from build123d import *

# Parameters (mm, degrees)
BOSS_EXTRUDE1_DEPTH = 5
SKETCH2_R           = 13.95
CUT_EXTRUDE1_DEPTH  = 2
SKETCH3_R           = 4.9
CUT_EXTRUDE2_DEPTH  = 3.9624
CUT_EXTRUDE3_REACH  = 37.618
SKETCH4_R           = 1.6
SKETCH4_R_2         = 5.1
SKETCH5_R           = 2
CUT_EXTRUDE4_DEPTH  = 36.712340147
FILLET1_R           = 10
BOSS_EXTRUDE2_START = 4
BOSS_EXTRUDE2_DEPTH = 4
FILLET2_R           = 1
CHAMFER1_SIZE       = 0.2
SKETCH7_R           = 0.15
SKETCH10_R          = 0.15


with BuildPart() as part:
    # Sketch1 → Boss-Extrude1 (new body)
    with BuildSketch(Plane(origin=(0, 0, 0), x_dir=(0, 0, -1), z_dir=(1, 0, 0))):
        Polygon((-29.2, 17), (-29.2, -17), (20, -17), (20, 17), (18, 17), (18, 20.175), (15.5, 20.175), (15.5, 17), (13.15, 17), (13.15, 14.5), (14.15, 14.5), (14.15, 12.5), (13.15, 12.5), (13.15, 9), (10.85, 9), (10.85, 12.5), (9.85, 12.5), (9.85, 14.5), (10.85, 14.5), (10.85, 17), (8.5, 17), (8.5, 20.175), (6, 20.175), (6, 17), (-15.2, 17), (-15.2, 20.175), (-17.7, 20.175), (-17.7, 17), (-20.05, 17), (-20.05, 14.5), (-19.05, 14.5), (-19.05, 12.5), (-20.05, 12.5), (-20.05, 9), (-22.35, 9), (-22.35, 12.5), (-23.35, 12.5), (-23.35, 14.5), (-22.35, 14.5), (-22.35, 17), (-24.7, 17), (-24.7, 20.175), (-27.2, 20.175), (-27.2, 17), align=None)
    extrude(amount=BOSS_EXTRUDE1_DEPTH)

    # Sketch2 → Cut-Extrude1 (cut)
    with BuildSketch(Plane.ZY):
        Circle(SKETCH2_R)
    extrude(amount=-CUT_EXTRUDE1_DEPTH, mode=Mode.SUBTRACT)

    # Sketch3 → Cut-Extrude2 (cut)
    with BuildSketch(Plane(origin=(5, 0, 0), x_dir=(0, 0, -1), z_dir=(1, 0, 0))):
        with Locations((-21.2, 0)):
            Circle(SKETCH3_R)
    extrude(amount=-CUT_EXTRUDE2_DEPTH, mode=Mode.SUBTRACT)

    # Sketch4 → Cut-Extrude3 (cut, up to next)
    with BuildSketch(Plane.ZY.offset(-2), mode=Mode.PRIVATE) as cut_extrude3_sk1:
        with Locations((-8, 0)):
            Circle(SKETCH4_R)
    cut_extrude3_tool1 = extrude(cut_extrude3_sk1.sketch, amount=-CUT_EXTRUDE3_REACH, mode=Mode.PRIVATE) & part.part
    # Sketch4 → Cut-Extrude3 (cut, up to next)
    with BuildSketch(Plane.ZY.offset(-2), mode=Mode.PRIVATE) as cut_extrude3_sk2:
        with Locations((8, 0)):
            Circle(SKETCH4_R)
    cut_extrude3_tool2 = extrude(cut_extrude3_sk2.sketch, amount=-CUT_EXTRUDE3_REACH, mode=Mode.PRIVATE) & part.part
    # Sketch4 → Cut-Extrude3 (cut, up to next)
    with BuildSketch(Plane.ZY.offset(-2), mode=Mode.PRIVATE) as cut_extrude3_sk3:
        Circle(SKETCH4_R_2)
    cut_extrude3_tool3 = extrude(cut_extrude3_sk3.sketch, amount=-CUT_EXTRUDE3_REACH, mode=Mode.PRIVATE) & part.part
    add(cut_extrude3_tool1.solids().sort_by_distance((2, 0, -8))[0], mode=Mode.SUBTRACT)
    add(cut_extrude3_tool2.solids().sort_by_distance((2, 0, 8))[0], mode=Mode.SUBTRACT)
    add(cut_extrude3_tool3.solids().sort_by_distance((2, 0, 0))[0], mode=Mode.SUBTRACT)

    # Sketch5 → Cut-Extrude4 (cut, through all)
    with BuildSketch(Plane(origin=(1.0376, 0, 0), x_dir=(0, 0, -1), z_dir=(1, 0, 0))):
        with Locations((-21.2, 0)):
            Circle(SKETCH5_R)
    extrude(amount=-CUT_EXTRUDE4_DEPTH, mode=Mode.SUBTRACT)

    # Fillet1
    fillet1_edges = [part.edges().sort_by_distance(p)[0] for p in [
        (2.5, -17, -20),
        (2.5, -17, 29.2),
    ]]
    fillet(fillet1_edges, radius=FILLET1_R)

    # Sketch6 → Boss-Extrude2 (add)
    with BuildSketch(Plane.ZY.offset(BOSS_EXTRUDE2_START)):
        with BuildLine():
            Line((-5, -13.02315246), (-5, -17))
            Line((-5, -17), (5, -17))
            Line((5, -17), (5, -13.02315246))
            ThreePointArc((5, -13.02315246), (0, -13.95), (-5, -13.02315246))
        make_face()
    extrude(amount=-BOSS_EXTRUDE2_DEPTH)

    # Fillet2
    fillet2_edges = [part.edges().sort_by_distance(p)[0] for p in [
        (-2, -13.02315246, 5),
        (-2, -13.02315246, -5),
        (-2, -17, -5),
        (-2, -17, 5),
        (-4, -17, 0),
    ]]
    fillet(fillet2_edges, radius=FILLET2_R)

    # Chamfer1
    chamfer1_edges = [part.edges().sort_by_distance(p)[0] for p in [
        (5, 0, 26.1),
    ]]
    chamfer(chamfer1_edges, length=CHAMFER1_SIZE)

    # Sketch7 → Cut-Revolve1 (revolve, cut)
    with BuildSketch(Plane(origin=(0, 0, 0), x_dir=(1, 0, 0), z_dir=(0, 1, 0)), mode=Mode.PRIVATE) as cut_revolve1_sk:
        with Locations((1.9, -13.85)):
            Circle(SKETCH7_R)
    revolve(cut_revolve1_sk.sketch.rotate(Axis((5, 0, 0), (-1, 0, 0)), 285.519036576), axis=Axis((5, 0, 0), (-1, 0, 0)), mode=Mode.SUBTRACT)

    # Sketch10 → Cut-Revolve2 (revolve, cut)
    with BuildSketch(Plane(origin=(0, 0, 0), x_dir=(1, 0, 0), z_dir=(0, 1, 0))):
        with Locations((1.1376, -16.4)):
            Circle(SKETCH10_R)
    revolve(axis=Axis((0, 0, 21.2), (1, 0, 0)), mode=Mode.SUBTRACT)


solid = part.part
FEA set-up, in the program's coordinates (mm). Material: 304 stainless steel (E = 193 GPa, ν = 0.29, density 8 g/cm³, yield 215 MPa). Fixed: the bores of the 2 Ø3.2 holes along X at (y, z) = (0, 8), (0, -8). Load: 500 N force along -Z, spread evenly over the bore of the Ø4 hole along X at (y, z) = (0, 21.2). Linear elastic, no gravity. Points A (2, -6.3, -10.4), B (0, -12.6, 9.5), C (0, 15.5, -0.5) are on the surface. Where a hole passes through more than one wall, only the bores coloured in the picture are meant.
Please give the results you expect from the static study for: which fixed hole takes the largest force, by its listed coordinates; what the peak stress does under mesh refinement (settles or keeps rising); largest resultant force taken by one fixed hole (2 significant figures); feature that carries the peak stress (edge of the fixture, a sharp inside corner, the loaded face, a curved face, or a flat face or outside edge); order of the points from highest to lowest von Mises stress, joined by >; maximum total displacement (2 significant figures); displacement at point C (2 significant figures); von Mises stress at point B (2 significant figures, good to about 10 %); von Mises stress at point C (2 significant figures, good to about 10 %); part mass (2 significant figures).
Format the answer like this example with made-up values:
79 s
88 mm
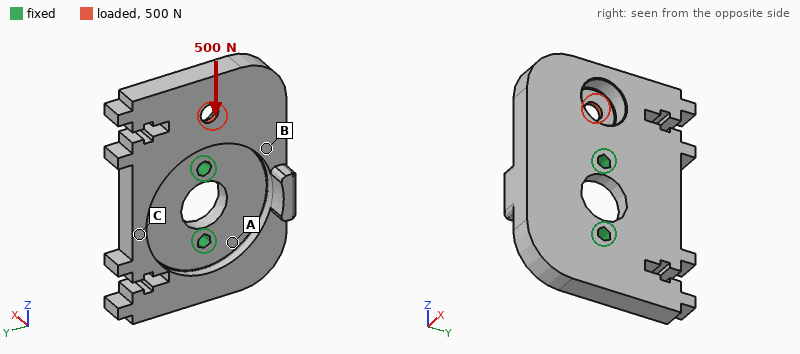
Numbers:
(0, 8)
keeps rising
370 N
edge of the fixture
B > C > A
11 µm
1.7 µm
15 MPa
10 MPa
51 g
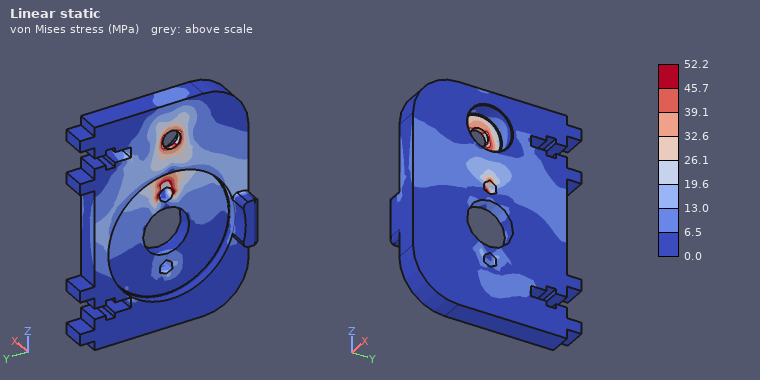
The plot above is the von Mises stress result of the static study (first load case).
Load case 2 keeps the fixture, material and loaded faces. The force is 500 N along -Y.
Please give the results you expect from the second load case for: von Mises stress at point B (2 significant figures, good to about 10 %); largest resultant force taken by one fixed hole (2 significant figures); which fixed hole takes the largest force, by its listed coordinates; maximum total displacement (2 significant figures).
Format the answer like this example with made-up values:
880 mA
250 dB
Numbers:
5.3 MPa
800 N
(0, 8)
14 µm
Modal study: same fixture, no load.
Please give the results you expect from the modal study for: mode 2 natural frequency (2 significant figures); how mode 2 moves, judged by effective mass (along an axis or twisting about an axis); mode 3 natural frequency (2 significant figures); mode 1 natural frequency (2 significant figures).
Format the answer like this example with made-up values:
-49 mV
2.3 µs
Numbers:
4800 Hz
along X
7200 Hz
4300 Hz
